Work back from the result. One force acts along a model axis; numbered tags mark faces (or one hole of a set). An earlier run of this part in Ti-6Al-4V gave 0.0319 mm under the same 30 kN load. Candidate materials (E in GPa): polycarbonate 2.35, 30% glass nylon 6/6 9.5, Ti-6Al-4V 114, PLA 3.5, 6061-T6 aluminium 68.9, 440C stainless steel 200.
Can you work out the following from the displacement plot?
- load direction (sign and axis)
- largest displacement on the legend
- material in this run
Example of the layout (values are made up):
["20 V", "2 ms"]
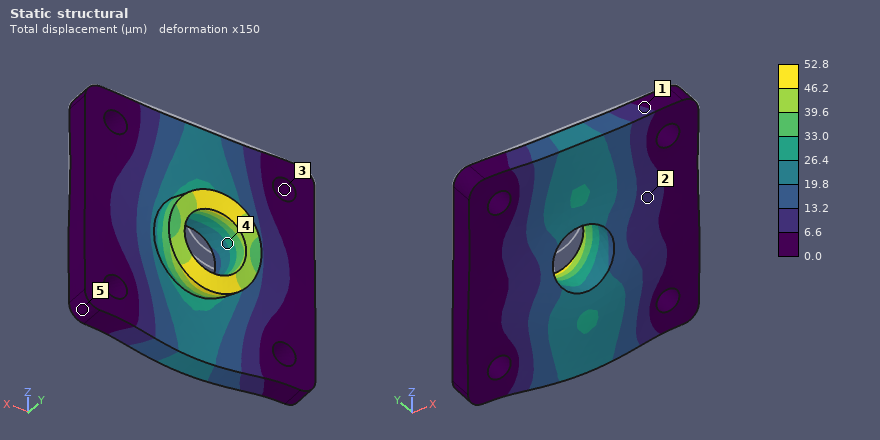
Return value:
["-Z", "52.8 µm", "6061-T6 aluminium"]
